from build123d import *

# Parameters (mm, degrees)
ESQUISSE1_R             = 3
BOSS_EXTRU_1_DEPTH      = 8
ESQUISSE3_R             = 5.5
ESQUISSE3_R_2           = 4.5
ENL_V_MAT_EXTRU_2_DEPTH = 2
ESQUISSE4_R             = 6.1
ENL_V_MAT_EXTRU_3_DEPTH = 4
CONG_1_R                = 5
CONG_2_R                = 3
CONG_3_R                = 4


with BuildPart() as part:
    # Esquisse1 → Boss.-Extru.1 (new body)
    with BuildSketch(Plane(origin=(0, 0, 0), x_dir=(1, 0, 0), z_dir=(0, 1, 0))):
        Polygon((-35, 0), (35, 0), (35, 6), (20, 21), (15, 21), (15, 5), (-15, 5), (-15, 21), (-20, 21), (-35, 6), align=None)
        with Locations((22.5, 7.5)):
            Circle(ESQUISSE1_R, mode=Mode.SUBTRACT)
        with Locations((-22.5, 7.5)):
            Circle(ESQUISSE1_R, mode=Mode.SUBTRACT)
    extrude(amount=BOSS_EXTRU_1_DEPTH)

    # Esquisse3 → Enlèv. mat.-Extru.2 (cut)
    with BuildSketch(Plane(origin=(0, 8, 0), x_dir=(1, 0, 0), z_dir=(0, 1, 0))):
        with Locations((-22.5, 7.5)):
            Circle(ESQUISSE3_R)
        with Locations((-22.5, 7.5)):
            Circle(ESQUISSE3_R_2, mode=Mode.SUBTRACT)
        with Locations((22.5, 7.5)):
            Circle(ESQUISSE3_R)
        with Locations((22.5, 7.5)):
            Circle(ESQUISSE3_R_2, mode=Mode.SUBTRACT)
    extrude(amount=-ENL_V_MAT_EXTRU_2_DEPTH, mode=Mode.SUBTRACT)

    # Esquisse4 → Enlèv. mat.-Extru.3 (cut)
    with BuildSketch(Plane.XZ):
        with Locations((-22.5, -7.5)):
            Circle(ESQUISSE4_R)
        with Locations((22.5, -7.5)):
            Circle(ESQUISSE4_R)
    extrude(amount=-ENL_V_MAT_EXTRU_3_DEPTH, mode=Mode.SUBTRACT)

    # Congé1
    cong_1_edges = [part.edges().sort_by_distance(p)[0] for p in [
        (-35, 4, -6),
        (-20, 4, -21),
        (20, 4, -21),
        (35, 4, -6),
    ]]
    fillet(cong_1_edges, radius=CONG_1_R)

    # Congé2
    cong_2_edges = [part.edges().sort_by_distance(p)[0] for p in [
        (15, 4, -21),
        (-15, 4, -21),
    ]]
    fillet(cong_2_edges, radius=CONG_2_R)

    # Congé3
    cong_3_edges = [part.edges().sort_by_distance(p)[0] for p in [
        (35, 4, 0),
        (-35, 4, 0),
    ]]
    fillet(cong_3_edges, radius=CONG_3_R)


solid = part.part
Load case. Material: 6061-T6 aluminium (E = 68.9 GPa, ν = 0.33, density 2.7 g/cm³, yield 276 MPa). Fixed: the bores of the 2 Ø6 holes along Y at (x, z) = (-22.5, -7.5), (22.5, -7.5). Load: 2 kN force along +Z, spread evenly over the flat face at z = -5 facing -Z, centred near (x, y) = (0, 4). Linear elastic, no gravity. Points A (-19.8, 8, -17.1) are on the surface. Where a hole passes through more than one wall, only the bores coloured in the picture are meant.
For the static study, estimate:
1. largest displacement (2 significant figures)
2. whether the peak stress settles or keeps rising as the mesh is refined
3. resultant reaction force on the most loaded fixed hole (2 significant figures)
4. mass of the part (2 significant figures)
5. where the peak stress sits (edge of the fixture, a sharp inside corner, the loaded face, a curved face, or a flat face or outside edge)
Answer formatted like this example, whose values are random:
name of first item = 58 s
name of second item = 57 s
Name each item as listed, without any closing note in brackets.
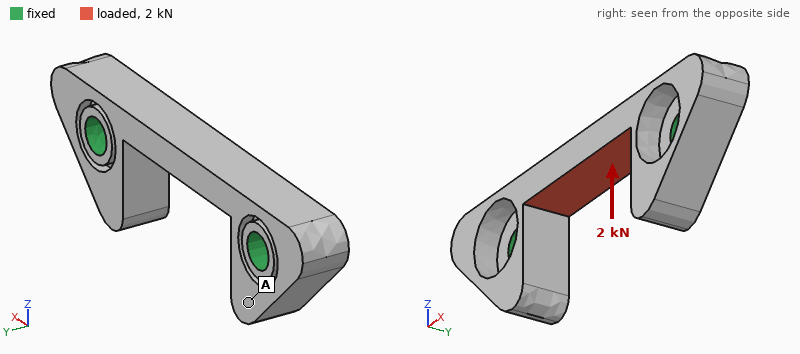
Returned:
largest displacement = 83 µm
whether the peak stress settles or keeps rising as the mesh is refined = keeps rising
resultant reaction force on the most loaded fixed hole = 1.2 kN
mass of the part = 13 g
where the peak stress sits = edge of the fixture
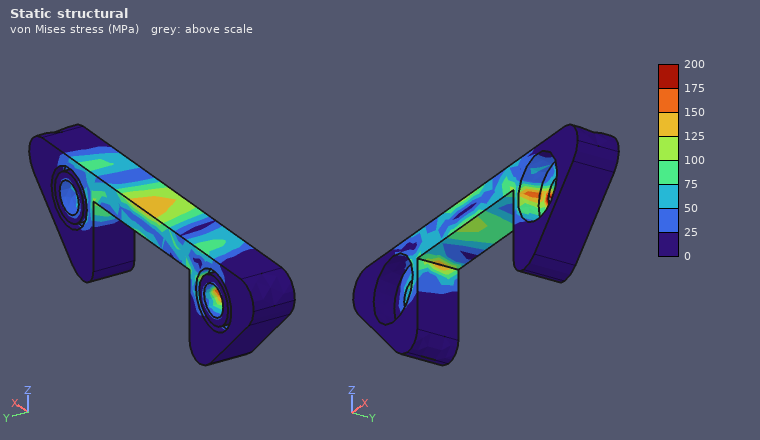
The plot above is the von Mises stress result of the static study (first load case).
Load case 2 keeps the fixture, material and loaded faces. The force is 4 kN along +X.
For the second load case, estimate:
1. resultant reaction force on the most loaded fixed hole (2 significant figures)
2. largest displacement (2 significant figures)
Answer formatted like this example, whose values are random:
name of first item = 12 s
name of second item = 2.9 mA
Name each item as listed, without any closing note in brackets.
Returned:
resultant reaction force on the most loaded fixed hole = 2.0 kN
largest displacement = 24 µm
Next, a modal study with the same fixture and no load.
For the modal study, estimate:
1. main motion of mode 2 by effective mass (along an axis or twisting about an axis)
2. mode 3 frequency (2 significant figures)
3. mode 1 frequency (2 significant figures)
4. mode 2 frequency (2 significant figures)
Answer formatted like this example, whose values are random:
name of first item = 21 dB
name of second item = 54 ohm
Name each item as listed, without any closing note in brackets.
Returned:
main motion of mode 2 by effective mass = along Z
mode 3 frequency = 17 kHz
mode 1 frequency = 13 kHz
mode 2 frequency = 16 kHz
